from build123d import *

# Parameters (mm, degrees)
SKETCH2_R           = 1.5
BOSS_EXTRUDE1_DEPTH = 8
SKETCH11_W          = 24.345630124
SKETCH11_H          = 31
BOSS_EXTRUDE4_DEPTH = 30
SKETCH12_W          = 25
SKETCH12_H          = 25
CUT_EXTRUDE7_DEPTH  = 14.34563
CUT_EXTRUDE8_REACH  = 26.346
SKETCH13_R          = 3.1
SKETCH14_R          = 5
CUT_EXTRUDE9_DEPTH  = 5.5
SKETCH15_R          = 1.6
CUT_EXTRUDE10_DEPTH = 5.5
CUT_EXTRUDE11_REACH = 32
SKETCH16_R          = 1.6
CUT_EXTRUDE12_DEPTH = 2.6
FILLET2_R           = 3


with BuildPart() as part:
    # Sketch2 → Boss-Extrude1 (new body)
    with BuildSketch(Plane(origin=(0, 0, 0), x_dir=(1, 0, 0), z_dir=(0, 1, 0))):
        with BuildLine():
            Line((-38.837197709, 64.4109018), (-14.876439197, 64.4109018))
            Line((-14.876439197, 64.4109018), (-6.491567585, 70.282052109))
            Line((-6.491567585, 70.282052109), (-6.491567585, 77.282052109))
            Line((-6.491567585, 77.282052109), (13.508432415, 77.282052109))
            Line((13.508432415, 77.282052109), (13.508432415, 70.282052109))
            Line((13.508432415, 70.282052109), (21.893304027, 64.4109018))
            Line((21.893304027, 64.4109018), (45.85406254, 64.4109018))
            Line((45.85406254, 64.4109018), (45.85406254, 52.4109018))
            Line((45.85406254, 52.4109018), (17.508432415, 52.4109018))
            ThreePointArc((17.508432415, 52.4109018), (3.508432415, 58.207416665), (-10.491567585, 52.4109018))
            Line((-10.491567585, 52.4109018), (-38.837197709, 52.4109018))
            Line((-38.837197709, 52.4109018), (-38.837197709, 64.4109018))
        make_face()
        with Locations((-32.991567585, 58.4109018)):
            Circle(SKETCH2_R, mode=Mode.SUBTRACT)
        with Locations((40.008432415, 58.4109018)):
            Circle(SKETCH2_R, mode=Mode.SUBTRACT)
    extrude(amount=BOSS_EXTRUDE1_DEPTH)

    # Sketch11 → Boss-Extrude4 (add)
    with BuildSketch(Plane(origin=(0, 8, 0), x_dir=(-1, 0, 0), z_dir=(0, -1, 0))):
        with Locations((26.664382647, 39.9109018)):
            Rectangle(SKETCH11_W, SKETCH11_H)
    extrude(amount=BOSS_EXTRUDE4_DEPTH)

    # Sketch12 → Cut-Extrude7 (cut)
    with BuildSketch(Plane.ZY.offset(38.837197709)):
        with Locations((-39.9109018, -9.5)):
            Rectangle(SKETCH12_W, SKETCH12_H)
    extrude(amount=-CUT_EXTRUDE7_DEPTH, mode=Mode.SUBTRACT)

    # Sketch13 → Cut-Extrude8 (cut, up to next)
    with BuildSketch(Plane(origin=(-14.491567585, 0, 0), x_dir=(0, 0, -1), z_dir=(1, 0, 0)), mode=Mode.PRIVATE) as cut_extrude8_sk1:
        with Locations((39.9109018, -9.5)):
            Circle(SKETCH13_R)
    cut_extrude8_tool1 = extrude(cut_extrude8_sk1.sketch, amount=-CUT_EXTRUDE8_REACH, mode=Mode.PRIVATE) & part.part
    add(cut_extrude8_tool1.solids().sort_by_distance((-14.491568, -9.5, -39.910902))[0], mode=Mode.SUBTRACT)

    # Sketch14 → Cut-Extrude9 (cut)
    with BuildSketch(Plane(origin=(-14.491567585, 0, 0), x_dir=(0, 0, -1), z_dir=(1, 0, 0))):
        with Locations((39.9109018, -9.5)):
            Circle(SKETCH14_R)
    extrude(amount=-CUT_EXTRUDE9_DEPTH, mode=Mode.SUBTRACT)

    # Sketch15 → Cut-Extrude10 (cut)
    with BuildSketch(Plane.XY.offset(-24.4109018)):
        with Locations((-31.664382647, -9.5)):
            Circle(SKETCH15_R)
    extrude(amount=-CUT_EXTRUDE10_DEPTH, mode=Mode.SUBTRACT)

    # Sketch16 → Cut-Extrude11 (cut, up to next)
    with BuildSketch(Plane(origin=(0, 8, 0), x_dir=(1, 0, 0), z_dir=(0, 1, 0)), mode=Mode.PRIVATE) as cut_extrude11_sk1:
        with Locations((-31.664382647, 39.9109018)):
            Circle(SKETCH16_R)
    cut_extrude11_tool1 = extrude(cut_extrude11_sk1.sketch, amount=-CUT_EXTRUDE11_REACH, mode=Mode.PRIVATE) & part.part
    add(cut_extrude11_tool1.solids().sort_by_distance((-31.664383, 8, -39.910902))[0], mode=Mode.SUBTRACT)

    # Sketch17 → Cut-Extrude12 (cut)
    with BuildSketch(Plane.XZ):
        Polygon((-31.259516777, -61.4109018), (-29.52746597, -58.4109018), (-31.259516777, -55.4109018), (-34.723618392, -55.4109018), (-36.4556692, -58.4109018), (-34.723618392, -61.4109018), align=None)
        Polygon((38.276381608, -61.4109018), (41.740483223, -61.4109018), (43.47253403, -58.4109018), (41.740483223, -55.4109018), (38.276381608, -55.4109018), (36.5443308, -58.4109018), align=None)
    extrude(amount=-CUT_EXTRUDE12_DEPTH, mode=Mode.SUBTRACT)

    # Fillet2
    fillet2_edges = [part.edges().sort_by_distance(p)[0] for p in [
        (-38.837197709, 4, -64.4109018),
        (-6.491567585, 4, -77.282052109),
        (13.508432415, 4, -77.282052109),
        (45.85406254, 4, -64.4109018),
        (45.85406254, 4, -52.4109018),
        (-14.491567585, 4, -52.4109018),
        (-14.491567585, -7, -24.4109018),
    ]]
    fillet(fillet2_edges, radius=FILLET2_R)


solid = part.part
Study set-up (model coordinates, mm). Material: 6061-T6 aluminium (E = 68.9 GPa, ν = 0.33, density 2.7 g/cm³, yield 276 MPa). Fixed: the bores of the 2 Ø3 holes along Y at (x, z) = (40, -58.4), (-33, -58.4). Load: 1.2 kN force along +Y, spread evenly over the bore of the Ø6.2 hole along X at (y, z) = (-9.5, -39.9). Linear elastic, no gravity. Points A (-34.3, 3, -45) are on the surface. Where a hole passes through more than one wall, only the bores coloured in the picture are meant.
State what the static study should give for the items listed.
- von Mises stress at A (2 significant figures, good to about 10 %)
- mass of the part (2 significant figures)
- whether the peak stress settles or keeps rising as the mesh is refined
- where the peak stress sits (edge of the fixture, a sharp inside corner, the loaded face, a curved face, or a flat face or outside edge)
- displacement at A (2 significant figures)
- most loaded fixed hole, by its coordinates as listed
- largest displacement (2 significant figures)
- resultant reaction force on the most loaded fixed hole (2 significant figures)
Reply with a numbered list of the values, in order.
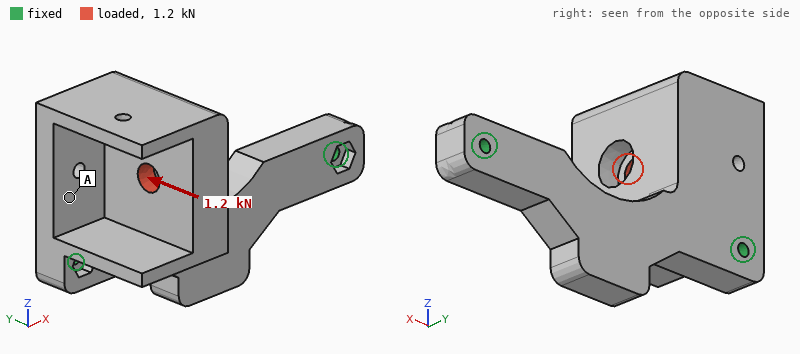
1. 30 MPa
2. 59 g
3. keeps rising
4. edge of the fixture
5. 0.072 mm
6. (-33, -58.4)
7. 0.34 mm
8. 1.1 kN
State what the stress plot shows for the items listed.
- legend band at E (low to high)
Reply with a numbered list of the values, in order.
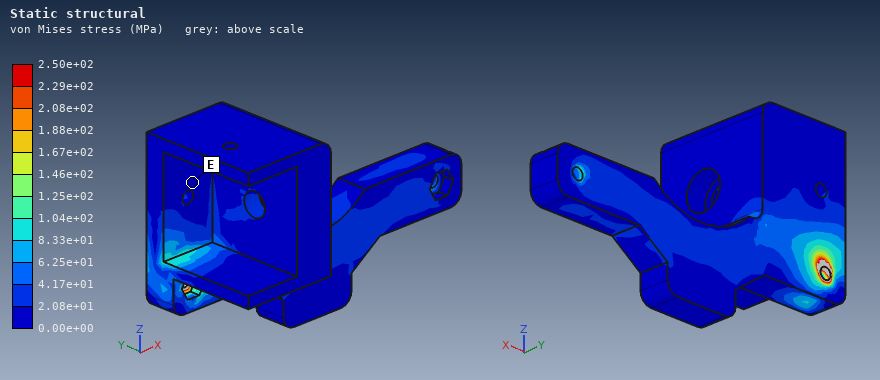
1. 0.00e+00 to 2.08e+01 MPa
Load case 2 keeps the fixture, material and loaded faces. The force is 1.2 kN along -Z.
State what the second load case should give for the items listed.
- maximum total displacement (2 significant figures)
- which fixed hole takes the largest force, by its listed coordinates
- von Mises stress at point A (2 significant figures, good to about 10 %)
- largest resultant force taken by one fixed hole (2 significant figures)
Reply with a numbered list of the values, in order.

1. 0.27 mm
2. (-33, -58.4)
3. 29 MPa
4. 1.1 kN
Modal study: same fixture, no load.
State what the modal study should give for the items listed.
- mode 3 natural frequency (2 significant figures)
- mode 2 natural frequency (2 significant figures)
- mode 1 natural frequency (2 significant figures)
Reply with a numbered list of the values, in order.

1. 4500 Hz
2. 2900 Hz
3. 1800 Hz
